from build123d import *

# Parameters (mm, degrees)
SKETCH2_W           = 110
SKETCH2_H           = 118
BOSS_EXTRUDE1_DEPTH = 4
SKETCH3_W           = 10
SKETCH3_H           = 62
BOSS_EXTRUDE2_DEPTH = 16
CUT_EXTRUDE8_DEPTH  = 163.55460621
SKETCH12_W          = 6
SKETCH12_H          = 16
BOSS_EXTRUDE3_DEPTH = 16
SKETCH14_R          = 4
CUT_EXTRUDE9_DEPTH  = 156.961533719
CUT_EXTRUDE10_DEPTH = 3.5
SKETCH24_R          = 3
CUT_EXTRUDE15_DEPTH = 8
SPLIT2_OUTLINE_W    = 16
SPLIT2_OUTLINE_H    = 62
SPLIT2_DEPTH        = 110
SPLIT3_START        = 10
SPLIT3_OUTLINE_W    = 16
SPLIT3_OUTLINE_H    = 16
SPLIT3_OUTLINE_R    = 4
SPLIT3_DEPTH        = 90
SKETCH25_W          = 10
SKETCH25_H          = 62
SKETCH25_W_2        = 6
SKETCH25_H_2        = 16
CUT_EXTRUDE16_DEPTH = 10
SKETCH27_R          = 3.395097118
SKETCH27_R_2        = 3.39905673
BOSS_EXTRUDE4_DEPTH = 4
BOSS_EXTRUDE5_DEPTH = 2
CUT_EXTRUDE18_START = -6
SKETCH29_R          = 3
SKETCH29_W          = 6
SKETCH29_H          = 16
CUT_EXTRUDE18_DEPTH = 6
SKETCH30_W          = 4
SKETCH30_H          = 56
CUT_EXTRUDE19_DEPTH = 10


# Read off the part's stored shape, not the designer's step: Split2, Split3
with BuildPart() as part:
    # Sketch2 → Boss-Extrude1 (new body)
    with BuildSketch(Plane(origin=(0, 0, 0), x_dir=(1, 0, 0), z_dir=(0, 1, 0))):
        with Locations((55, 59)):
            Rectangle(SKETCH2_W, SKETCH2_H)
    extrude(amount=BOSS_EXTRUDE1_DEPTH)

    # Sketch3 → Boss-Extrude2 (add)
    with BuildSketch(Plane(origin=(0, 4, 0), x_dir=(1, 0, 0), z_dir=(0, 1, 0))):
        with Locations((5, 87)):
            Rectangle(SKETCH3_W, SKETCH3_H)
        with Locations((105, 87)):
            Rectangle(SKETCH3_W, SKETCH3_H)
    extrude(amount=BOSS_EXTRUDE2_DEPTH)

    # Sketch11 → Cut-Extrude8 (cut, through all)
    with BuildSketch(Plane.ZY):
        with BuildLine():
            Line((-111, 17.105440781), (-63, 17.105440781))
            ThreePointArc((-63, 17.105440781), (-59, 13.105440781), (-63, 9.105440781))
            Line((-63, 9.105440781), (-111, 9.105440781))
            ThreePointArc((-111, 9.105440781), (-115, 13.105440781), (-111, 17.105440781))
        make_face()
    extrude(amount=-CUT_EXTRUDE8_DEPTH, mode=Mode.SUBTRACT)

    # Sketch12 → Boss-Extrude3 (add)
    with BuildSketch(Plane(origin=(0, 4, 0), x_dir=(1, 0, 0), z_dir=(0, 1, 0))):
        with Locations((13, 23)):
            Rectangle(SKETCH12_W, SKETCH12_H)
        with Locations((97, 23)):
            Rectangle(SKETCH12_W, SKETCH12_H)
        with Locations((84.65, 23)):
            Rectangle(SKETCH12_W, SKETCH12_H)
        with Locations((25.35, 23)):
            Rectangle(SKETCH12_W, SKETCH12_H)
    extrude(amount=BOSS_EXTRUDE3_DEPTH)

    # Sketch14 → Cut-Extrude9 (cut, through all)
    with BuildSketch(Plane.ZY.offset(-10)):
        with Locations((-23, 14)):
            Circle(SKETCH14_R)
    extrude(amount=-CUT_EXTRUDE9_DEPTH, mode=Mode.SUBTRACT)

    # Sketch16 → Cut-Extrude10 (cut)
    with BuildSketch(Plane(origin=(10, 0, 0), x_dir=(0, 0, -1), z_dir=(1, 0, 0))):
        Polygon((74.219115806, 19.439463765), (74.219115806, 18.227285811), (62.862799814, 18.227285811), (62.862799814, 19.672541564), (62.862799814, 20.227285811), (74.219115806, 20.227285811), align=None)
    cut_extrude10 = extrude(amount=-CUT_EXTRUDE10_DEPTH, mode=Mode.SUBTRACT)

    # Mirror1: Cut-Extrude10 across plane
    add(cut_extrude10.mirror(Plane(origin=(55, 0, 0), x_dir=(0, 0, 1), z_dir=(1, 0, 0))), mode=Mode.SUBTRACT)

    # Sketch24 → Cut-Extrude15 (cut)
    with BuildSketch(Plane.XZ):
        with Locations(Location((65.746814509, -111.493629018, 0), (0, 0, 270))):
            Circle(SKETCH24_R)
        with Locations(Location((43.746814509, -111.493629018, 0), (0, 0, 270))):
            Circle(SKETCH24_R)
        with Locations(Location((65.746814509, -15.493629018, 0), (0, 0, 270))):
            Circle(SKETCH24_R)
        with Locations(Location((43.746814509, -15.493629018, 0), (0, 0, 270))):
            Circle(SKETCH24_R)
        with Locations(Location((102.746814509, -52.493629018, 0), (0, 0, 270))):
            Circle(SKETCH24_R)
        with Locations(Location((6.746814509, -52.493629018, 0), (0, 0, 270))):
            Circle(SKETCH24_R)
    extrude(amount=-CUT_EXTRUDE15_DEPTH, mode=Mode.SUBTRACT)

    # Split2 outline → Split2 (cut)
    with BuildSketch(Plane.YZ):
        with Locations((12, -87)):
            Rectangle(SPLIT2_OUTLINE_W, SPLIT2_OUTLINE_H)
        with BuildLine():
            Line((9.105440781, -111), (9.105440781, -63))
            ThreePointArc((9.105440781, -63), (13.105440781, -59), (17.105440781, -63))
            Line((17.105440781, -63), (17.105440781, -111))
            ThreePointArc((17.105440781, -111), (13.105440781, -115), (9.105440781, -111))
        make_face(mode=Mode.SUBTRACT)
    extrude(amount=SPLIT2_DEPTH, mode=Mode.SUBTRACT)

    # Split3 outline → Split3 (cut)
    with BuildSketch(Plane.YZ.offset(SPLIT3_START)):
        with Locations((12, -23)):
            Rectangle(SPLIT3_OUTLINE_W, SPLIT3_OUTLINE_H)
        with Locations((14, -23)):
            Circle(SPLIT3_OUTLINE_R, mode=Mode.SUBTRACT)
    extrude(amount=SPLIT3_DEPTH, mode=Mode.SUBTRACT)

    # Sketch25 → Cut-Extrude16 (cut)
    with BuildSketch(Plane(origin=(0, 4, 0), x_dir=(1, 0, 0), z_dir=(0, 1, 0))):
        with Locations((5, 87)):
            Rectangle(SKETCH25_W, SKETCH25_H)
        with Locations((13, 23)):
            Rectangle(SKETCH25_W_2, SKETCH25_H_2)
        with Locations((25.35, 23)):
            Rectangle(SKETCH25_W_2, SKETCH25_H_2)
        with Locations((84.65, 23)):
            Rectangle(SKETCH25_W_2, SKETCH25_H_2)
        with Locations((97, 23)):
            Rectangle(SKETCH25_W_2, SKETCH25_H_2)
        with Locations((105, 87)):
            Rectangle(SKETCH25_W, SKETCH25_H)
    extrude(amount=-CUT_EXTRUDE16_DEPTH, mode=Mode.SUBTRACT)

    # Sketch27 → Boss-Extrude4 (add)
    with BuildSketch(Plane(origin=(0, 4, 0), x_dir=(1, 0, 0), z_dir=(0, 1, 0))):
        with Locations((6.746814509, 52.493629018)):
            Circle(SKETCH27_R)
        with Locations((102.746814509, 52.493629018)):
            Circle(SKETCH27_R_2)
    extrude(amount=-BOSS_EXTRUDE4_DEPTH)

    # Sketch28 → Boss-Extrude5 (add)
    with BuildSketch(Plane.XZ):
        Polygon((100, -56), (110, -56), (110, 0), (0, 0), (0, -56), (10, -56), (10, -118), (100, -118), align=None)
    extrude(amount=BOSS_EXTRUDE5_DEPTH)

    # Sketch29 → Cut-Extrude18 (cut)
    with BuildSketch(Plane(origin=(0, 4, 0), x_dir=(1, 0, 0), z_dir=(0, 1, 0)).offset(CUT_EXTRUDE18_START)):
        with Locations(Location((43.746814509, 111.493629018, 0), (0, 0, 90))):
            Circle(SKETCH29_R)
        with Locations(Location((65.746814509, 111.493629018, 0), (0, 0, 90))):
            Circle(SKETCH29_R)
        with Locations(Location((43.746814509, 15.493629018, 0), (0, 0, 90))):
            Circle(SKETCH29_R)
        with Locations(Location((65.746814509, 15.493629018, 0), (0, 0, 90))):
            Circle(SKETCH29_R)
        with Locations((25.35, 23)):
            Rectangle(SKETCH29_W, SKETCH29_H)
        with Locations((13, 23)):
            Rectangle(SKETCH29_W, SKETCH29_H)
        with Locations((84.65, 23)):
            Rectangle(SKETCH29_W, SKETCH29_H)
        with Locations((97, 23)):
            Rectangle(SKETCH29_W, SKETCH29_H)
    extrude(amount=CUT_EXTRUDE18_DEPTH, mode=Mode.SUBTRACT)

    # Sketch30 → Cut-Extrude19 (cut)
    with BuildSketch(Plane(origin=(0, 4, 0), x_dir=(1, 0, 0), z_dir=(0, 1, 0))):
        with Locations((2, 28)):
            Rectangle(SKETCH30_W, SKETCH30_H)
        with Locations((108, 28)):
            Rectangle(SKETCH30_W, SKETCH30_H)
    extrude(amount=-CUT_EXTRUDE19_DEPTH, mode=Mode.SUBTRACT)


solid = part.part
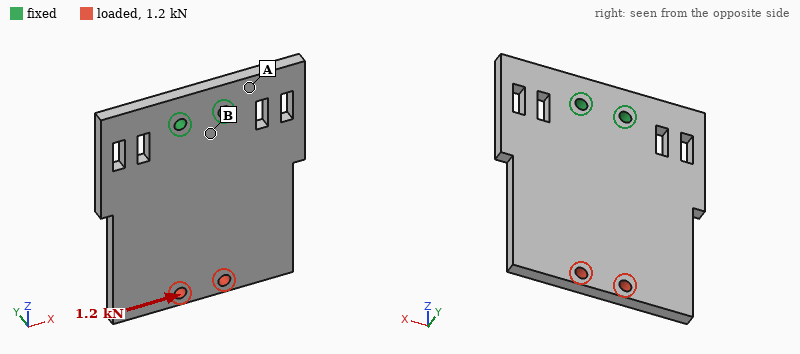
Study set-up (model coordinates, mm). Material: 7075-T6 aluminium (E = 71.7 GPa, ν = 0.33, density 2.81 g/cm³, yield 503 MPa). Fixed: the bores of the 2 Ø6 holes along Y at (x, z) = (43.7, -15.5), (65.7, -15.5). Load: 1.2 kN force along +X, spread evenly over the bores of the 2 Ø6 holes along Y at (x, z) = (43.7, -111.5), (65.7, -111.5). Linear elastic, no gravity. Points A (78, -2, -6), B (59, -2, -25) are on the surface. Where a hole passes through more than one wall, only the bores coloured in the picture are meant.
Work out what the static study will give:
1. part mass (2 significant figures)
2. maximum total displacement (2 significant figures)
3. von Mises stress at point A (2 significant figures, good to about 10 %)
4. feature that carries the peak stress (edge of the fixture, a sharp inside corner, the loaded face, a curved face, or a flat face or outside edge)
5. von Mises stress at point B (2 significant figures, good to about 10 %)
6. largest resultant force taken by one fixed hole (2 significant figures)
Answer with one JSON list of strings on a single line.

["180 g", "99 µm", "9.8 MPa", "edge of the fixture", "27 MPa", "4.3 kN"]
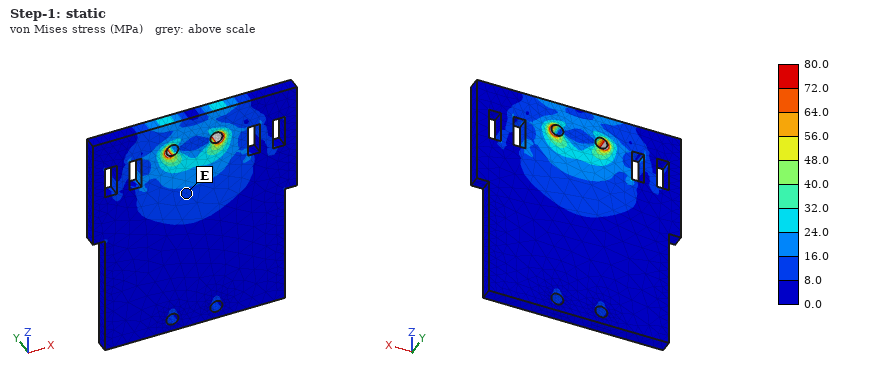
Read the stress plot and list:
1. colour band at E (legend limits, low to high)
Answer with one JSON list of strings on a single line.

["8.0 to 16.0 MPa"]
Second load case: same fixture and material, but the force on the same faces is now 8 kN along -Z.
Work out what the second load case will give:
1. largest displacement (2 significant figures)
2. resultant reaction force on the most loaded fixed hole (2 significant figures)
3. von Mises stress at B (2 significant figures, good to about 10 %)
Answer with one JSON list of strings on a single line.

["39 µm", "4.0 kN", "22 MPa"]
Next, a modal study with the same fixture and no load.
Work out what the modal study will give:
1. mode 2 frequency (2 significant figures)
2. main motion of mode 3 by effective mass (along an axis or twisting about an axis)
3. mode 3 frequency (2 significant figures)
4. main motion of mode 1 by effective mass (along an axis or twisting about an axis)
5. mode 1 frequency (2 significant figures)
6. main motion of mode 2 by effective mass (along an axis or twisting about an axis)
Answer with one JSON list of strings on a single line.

["1000 Hz", "along X", "2300 Hz", "along Y", "440 Hz", "twisting about Z"]
